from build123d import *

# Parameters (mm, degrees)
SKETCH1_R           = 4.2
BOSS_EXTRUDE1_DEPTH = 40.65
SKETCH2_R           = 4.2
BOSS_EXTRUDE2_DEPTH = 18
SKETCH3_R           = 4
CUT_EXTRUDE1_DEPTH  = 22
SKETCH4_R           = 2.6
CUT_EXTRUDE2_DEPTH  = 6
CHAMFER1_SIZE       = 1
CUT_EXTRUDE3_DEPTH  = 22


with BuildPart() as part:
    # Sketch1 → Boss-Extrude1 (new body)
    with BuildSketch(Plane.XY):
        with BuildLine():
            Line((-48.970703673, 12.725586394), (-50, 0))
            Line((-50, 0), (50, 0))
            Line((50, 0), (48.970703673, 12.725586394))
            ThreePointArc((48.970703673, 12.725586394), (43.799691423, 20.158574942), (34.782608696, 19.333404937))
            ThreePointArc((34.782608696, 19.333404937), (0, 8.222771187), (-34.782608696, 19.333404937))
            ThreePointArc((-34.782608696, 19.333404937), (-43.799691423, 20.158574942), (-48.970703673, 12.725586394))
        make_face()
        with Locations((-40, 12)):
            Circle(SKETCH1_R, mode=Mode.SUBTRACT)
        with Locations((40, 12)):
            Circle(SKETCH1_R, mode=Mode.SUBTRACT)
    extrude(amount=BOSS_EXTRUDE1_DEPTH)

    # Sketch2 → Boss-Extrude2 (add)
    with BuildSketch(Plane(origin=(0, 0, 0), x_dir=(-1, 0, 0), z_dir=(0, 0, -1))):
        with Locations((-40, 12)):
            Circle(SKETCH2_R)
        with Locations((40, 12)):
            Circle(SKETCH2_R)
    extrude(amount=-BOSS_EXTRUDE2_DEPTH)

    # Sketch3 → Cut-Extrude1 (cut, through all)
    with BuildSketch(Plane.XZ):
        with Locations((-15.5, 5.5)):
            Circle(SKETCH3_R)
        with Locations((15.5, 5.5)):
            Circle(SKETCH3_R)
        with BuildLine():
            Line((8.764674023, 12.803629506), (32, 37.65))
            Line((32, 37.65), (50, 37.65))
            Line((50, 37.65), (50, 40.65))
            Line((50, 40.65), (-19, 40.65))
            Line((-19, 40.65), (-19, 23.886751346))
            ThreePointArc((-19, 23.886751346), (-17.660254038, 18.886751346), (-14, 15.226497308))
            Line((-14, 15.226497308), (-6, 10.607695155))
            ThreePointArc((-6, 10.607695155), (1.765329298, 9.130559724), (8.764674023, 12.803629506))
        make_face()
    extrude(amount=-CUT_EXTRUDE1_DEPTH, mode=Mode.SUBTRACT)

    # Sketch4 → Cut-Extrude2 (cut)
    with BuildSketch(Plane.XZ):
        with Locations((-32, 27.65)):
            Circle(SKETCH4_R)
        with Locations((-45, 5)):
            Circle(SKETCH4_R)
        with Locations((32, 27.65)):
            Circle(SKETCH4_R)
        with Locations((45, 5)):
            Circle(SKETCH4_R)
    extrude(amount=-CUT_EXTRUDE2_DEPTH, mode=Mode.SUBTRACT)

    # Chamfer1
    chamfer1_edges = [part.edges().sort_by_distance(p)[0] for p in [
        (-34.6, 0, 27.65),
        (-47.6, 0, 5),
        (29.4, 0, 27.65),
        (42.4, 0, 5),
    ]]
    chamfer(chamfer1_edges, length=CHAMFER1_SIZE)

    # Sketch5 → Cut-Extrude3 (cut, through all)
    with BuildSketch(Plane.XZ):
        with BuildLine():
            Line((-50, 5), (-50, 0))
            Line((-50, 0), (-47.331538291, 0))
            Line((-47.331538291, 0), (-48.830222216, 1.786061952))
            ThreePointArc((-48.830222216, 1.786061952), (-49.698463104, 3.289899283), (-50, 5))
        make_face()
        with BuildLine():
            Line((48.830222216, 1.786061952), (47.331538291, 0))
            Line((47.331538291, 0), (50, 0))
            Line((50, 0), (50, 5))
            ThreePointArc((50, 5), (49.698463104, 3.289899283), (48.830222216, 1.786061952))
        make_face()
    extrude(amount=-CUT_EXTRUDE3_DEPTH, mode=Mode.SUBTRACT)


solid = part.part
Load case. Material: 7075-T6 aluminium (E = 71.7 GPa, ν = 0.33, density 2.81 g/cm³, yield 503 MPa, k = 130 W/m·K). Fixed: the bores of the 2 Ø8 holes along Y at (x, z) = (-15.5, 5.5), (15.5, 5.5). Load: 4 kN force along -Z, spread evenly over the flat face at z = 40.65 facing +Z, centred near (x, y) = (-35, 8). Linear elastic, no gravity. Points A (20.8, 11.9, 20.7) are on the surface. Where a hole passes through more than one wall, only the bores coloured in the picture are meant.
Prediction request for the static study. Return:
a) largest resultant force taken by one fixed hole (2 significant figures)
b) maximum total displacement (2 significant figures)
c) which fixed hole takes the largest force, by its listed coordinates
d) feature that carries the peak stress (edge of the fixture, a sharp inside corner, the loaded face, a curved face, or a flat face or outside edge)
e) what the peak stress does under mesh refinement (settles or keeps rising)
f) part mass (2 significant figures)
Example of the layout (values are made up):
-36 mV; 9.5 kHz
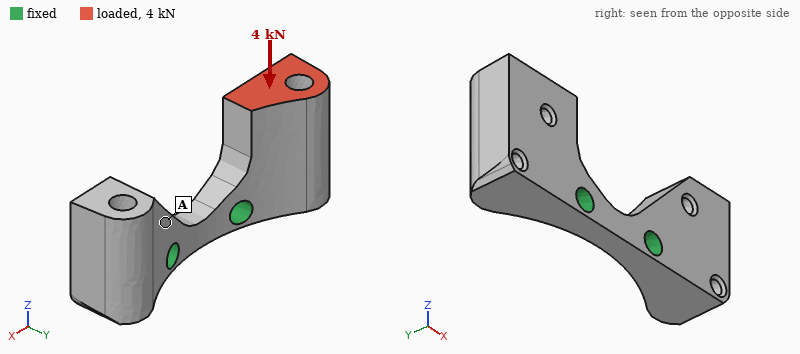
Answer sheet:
4.3 kN; 0.13 mm; (-15.5, 5.5); edge of the fixture; keeps rising; 110 g
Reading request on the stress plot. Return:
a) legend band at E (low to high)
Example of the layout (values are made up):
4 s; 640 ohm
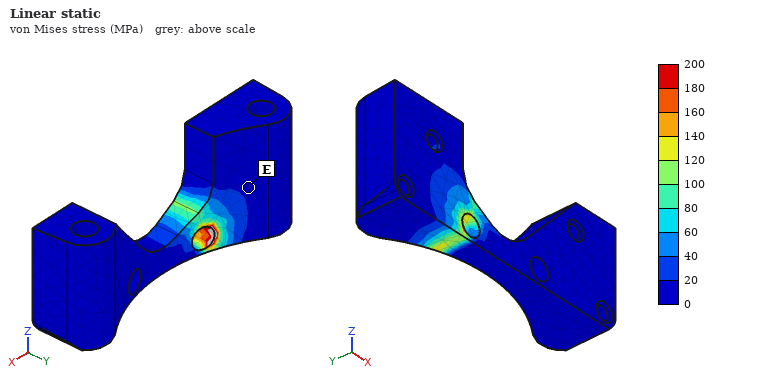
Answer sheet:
0 to 20 MPa
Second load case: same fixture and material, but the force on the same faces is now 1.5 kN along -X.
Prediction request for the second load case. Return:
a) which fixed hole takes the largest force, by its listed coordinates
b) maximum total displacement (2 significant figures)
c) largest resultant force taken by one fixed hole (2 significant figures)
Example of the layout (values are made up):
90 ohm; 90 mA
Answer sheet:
(-15.5, 5.5); 0.10 mm; 1.4 kN
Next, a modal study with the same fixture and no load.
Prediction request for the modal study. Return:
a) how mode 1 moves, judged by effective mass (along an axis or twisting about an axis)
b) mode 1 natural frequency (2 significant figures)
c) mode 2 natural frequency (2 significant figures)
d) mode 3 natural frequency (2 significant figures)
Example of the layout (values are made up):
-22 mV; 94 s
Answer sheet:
along Y; 3800 Hz; 4200 Hz; 4400 Hz
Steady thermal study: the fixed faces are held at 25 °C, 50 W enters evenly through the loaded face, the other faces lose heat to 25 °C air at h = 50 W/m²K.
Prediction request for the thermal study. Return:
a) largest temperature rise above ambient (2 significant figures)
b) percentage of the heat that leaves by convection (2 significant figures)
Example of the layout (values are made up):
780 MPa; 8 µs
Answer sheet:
40 K; 12 %
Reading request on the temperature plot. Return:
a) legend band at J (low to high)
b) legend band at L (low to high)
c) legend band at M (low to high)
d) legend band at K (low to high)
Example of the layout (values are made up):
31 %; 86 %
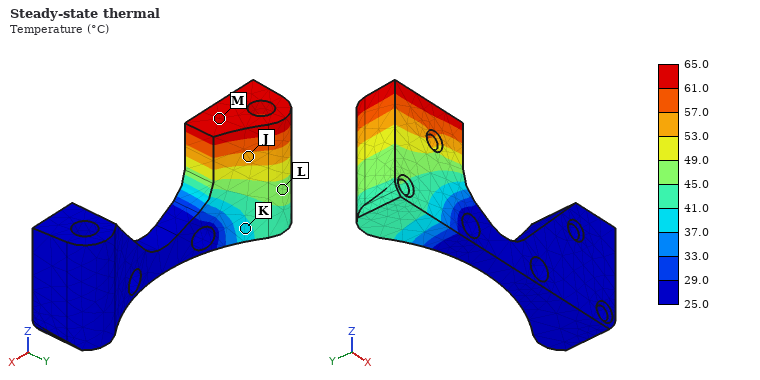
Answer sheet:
53.0 to 57.0 °C; 45.0 to 49.0 °C; 61.0 to 65.0 °C; 37.0 to 41.0 °C
